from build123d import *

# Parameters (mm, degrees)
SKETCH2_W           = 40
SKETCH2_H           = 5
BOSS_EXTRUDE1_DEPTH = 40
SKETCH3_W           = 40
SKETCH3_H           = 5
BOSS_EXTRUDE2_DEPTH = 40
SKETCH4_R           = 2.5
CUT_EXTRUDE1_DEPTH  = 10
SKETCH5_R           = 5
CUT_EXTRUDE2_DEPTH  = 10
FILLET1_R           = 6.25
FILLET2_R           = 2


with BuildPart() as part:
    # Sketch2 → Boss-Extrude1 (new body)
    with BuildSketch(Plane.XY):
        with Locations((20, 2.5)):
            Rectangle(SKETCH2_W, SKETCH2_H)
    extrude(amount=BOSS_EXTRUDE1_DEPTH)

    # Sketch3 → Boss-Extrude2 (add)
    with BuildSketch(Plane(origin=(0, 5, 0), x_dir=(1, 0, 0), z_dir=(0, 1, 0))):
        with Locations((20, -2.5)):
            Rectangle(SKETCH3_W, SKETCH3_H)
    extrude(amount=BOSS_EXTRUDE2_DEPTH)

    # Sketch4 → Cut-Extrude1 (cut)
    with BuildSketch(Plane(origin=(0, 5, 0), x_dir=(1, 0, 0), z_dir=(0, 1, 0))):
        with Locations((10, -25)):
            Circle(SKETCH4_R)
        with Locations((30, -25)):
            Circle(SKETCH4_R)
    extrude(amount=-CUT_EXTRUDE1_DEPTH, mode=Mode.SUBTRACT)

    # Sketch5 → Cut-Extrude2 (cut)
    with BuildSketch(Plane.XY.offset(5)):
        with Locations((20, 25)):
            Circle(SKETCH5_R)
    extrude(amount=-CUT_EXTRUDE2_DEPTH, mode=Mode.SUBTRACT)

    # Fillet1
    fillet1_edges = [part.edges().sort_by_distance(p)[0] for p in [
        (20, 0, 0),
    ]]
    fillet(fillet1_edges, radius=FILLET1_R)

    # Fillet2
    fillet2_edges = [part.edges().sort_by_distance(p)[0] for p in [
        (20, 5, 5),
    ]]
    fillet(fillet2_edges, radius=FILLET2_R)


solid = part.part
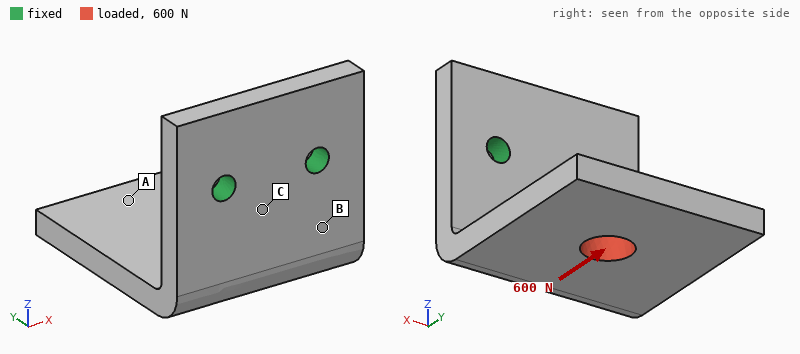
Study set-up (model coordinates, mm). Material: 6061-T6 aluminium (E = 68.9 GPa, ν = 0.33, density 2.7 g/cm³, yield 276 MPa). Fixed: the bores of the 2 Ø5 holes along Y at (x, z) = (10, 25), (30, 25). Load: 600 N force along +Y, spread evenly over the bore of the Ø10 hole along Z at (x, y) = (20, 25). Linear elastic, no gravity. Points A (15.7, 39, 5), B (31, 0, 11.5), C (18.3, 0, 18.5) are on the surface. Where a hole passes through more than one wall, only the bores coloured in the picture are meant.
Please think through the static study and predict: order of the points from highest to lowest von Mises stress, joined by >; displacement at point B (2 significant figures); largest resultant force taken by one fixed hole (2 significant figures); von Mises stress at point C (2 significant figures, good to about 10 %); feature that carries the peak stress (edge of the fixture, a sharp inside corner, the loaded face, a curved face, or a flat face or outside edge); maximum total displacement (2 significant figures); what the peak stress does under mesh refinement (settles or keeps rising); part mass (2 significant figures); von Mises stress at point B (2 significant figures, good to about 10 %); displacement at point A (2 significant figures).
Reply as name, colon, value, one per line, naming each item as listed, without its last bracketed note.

order of the points from highest to lowest von Mises stress, joined by >: C > B > A
displacement at point B: 0.034 mm
largest resultant force taken by one fixed hole: 300 N
von Mises stress at point C: 46 MPa
feature that carries the peak stress: edge of the fixture
maximum total displacement: 0.22 mm
what the peak stress does under mesh refinement: keeps rising
part mass: 41 g
von Mises stress at point B: 29 MPa
displacement at point A: 0.19 mm
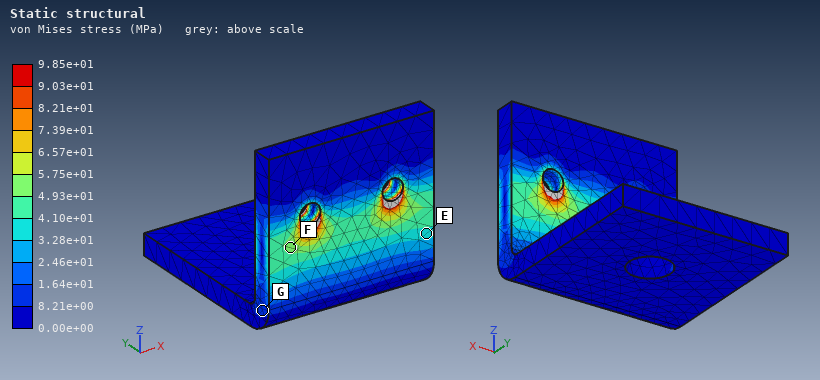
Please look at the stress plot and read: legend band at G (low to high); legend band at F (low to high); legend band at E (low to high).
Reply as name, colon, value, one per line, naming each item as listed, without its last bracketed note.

legend band at G: 8.21e+00 to 1.64e+01 MPa
legend band at F: 4.93e+01 to 5.75e+01 MPa
legend band at E: 3.28e+01 to 4.10e+01 MPa
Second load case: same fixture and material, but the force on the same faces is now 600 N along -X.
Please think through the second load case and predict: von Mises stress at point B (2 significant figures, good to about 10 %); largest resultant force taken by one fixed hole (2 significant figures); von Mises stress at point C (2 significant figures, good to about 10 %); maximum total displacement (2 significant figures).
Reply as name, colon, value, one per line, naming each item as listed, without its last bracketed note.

von Mises stress at point B: 33 MPa
largest resultant force taken by one fixed hole: 820 N
von Mises stress at point C: 23 MPa
maximum total displacement: 0.17 mm
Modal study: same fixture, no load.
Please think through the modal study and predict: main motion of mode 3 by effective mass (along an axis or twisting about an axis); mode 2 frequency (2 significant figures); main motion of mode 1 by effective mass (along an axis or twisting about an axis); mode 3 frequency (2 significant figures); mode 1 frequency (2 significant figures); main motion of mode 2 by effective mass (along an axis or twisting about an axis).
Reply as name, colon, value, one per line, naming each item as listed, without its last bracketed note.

main motion of mode 3 by effective mass: along Y
mode 2 frequency: 2400 Hz
main motion of mode 1 by effective mass: along Z
mode 3 frequency: 4300 Hz
mode 1 frequency: 1300 Hz
main motion of mode 2 by effective mass: along X
